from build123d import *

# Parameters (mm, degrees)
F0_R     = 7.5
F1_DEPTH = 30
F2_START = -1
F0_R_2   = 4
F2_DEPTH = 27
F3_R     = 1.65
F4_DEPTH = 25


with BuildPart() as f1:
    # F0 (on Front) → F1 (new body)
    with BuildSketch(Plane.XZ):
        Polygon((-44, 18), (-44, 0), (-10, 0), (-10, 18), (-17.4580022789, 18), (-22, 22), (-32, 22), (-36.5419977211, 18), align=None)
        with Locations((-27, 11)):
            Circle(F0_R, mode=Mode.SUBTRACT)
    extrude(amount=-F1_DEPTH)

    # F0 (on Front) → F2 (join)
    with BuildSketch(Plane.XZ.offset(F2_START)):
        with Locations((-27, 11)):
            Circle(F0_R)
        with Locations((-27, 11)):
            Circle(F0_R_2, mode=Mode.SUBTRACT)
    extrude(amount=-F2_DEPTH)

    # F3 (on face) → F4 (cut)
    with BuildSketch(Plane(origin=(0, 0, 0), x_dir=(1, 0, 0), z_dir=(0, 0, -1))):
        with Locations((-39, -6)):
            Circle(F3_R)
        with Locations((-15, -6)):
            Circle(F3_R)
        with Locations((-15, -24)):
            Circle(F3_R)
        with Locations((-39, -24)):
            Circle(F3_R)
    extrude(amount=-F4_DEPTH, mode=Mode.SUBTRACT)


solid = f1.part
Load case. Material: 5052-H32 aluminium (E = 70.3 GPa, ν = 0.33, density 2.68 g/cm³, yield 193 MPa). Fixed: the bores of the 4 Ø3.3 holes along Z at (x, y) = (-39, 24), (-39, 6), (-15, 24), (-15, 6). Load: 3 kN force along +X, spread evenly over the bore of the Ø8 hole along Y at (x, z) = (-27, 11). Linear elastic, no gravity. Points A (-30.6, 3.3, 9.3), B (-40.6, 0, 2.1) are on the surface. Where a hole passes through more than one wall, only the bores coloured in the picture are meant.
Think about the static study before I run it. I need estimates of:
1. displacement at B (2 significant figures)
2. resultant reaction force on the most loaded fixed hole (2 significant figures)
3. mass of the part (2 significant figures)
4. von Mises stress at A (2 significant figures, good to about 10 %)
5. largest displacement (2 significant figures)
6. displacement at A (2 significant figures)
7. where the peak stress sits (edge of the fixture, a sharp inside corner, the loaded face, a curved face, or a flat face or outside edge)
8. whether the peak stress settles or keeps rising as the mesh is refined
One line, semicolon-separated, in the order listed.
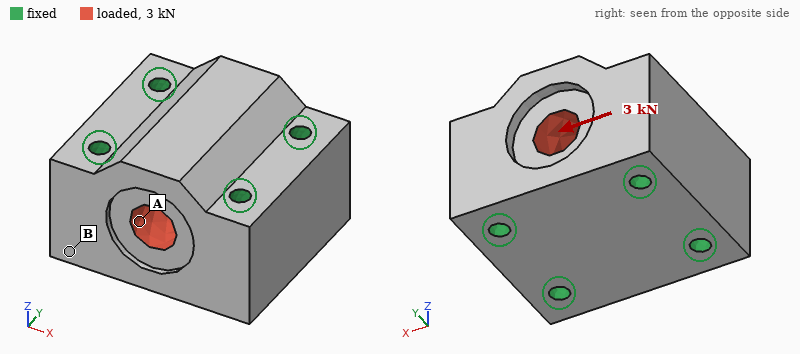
0.13 µm; 790 N; 47 g; 5.2 MPa; 0.85 µm; 0.51 µm; edge of the fixture; keeps rising
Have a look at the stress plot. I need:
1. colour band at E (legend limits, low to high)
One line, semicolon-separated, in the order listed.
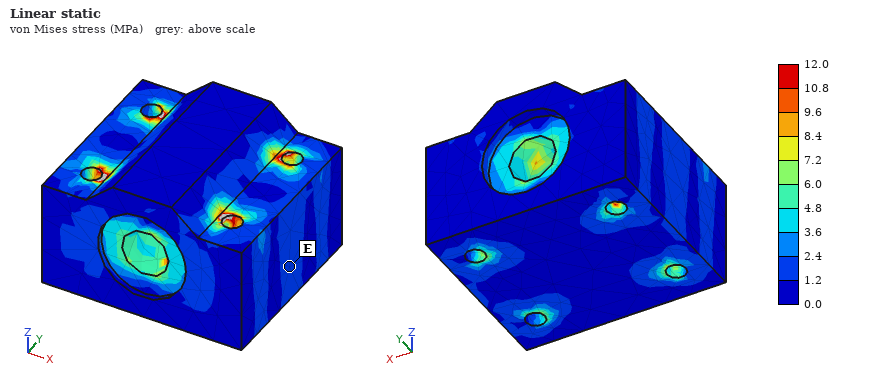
1.2 to 2.4 MPa
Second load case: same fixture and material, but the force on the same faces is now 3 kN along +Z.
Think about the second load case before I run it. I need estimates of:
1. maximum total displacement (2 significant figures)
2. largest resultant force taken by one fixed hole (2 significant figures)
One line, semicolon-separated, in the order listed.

1.6 µm; 780 N
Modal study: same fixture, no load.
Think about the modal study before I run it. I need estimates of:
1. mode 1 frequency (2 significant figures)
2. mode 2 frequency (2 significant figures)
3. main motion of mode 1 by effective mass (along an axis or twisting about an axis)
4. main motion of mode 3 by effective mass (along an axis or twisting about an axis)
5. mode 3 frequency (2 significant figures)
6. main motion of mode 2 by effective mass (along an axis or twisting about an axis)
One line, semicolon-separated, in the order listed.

52 kHz; 55 kHz; along Y; along Y; 62 kHz; along Z
